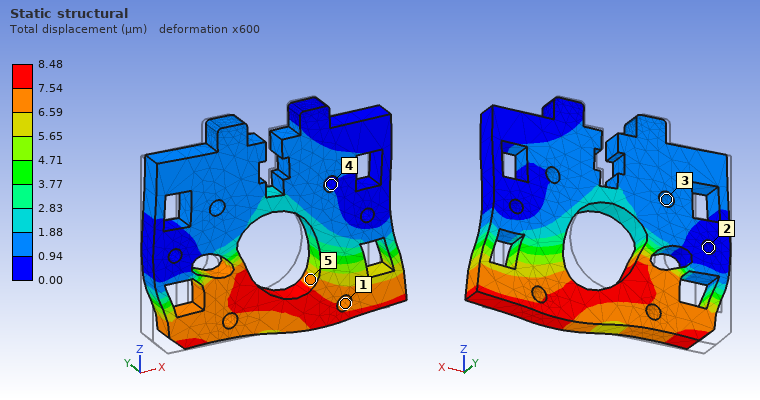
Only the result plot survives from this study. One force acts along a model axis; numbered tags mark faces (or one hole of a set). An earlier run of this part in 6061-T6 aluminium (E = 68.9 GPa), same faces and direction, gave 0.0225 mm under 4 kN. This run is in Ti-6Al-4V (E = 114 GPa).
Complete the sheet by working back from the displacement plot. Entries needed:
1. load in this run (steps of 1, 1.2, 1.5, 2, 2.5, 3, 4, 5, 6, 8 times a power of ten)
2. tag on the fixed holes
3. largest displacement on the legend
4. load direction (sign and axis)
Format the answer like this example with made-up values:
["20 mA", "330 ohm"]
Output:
["2.5 kN", "2", "8.48 µm", "+X"]
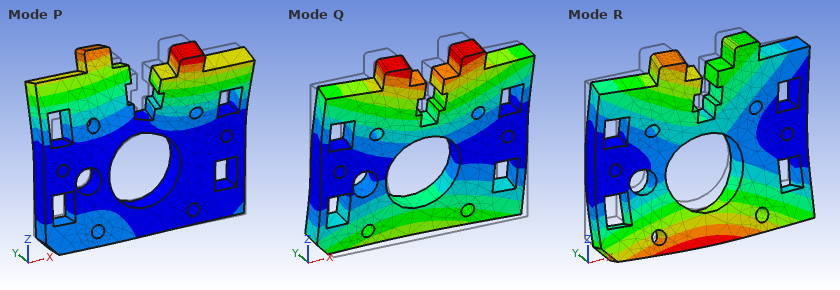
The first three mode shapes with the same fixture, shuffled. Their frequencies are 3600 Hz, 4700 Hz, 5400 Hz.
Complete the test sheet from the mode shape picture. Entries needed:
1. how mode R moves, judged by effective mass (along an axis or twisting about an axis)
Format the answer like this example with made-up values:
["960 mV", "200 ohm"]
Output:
["along Y"]
